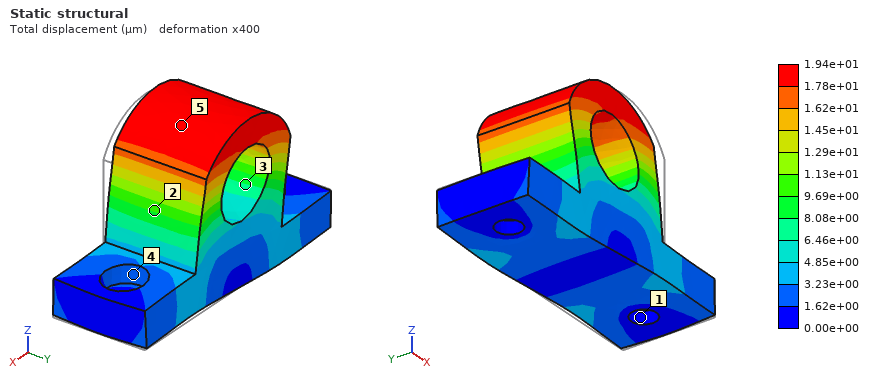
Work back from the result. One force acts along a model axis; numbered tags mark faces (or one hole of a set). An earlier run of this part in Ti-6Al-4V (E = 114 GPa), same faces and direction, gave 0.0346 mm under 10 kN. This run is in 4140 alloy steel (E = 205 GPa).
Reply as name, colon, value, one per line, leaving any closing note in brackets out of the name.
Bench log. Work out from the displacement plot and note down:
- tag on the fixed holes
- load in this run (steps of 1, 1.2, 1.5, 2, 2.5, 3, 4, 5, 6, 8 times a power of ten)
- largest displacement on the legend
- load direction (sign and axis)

tag on the fixed holes: 1
load in this run: 10 kN
largest displacement on the legend: 1.94e+01 µm
load direction: -X
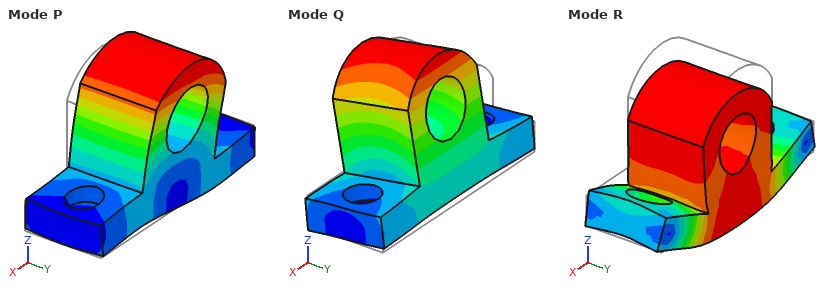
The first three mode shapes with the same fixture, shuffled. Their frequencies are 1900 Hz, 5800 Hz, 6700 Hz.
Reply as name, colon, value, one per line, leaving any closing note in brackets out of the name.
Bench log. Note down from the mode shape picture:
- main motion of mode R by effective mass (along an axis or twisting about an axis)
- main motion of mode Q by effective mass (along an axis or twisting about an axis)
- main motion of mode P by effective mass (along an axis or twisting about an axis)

main motion of mode R by effective mass: along Z
main motion of mode Q by effective mass: along Y
main motion of mode P by effective mass: along X
